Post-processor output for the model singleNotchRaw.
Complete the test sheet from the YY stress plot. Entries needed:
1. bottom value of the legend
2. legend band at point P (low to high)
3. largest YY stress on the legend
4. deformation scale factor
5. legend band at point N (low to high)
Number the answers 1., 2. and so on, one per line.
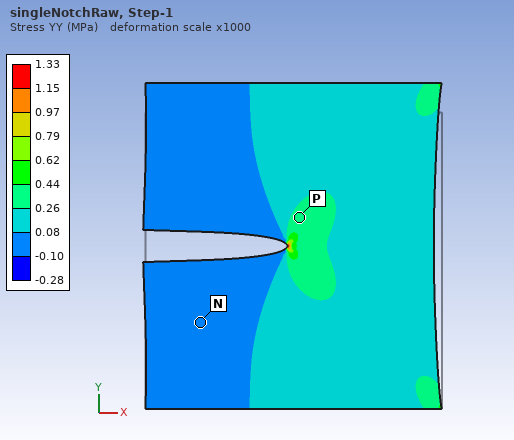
1. -0.28 MPa
2. 0.26 to 0.44 MPa
3. 1.33 MPa
4. 1000
5. -0.10 to 0.08 MPa
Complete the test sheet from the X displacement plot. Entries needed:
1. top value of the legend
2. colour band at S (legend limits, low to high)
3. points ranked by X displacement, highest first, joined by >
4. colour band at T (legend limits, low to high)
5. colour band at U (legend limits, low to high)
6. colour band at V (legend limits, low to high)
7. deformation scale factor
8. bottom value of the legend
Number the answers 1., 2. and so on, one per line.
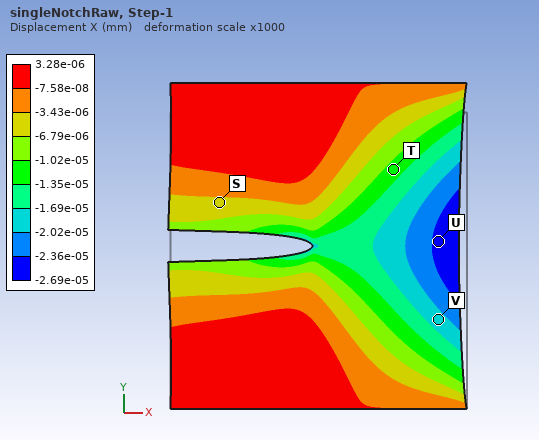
1. 3.28e-06 mm
2. -6.79e-06 to -3.43e-06 mm
3. S > T > V > U
4. -1.35e-05 to -1.02e-05 mm
5. -2.69e-05 to -2.36e-05 mm
6. -2.02e-05 to -1.69e-05 mm
7. 1000
8. -2.69e-05 mm
